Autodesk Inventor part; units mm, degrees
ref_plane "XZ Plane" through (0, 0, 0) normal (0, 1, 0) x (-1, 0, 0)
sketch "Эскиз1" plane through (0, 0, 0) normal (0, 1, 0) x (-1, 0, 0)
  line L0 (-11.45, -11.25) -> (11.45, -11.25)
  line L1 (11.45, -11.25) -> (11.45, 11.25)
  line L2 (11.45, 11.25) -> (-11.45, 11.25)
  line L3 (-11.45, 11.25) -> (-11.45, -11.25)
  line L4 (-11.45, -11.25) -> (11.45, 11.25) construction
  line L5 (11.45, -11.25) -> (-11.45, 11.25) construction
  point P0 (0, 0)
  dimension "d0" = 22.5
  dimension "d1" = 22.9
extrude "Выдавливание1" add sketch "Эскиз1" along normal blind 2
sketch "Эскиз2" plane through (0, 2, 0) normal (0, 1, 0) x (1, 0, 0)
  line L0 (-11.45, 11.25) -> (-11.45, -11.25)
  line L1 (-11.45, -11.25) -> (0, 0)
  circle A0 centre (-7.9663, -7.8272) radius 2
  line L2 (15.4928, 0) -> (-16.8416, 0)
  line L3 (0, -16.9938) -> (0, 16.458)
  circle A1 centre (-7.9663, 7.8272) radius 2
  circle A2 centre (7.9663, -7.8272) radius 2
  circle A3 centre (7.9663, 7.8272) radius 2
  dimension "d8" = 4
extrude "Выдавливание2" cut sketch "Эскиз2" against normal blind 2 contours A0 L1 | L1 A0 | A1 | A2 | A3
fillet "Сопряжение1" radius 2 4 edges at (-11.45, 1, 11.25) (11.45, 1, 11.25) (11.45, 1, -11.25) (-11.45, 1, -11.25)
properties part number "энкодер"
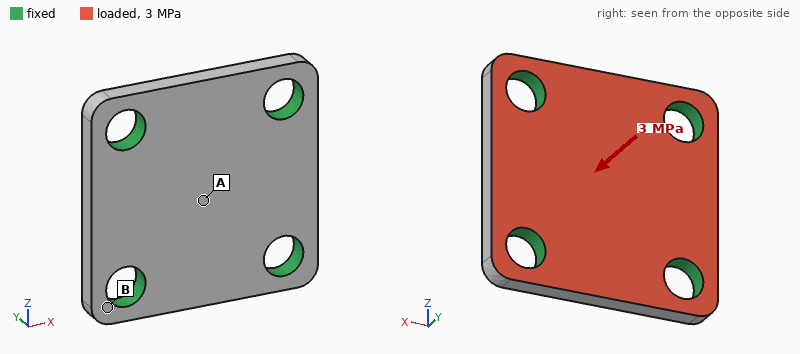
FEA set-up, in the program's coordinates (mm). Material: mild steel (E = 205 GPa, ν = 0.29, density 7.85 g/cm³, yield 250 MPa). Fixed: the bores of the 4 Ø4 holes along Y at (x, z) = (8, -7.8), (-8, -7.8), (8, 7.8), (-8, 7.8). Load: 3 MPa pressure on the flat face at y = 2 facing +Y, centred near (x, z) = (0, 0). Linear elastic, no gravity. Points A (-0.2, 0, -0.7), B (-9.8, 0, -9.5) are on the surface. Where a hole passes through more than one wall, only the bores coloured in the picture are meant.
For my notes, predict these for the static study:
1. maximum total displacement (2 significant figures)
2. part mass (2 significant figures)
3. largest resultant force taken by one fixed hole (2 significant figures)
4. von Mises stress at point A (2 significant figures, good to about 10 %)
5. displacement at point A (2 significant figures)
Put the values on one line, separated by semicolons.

4.8 µm; 7.2 g; 350 N; 37 MPa; 4.8 µm
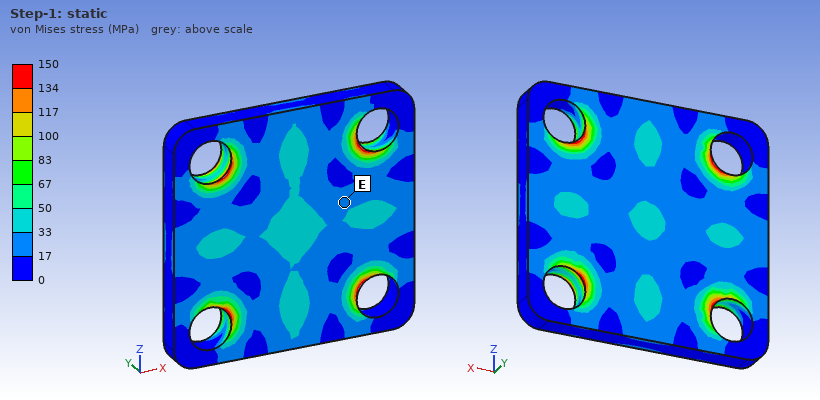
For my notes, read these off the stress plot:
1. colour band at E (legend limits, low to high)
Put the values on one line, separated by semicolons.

17 to 33 MPa
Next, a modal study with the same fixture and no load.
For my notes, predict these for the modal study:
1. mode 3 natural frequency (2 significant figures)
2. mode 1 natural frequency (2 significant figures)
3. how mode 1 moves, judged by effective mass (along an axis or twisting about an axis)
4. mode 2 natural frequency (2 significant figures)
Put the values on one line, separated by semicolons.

59 kHz; 39 kHz; along Y; 57 kHz
